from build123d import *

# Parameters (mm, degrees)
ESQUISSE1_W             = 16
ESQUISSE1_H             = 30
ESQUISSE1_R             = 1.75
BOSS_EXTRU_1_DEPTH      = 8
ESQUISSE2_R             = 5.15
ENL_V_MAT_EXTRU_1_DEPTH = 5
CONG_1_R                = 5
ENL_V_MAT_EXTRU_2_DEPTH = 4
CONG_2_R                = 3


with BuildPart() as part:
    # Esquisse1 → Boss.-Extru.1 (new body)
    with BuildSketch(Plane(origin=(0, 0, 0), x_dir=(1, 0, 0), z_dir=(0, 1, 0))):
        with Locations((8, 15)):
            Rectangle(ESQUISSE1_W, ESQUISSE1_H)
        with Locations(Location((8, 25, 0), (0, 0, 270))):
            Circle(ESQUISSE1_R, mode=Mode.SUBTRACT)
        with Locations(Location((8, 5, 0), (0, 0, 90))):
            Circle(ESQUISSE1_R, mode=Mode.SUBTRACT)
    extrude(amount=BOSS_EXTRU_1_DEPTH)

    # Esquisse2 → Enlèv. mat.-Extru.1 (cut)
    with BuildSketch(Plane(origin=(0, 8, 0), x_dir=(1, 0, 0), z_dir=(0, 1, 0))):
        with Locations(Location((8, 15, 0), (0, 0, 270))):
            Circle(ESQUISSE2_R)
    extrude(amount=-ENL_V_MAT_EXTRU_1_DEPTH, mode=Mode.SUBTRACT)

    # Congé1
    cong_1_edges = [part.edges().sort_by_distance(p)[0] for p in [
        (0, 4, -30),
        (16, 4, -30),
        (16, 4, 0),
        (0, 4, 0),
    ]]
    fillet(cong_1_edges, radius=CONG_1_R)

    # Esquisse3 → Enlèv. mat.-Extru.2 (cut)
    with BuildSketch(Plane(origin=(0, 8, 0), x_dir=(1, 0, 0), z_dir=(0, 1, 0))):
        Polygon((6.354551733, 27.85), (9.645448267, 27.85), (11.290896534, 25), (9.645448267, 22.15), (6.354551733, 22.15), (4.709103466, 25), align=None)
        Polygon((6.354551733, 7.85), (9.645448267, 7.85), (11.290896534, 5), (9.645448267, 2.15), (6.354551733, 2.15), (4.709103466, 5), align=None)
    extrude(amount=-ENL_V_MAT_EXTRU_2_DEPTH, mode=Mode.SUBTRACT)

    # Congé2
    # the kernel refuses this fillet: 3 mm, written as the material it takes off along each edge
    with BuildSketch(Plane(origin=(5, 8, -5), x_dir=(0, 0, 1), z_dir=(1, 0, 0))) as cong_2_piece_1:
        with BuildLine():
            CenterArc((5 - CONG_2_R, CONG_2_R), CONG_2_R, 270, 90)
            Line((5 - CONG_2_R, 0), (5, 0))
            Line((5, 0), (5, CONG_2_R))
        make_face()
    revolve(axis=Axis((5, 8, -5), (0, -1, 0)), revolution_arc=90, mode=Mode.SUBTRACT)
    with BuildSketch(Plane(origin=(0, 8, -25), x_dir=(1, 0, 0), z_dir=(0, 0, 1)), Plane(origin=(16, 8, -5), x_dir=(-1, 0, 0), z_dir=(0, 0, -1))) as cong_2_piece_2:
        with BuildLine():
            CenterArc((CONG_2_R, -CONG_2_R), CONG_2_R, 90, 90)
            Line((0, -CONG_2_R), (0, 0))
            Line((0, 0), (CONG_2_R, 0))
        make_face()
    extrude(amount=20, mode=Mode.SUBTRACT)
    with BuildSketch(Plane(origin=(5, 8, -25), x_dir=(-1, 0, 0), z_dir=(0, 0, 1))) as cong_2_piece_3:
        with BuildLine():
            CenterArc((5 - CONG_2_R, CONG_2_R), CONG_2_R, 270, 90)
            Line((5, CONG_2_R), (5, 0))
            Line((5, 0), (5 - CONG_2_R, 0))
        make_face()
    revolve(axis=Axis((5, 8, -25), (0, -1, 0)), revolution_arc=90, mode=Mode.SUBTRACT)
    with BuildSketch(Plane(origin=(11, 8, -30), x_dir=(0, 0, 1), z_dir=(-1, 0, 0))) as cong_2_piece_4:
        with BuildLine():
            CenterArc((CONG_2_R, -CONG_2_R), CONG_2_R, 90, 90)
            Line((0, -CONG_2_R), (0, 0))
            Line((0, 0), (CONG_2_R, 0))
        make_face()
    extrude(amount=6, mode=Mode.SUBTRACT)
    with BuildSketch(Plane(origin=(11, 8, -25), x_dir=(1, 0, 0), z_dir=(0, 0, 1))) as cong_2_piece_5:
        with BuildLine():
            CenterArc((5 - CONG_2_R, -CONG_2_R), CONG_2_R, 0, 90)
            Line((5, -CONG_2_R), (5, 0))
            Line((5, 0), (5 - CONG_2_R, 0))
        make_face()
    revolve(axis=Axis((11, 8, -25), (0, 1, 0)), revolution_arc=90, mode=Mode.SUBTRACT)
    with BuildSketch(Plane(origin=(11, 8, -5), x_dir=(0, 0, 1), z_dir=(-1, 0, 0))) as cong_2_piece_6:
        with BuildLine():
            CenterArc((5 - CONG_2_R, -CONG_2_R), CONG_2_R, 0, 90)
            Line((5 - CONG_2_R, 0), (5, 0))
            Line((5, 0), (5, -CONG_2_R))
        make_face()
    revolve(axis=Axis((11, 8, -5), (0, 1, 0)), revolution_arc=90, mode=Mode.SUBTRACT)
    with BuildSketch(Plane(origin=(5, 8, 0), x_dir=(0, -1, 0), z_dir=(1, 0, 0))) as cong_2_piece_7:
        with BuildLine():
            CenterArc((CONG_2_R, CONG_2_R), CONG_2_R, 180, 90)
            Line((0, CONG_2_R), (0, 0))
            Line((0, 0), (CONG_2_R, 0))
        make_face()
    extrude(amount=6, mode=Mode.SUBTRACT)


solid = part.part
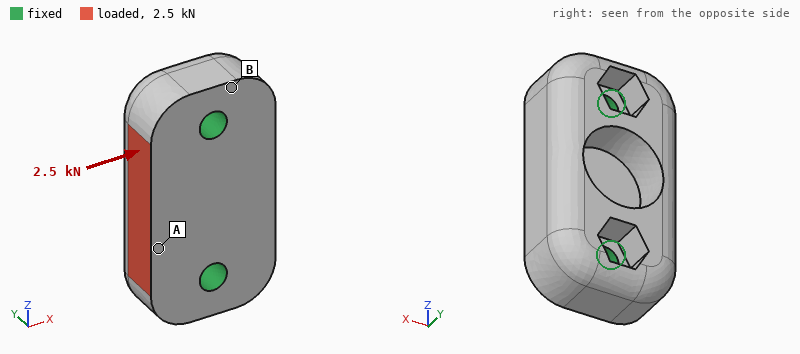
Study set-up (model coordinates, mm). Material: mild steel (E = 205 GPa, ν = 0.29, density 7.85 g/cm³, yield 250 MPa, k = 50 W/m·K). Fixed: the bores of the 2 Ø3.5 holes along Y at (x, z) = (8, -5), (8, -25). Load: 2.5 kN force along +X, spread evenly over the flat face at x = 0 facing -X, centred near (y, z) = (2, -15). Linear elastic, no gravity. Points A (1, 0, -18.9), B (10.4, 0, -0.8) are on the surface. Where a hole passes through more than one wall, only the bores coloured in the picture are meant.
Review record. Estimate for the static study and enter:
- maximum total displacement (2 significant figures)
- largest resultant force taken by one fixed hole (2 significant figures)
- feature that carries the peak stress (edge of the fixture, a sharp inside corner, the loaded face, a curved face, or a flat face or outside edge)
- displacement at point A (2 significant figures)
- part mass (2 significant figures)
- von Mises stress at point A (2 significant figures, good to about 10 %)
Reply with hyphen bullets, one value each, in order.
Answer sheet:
- 2.5 µm
- 1.3 kN
- edge of the fixture
- 1.8 µm
- 22 g
- 24 MPa
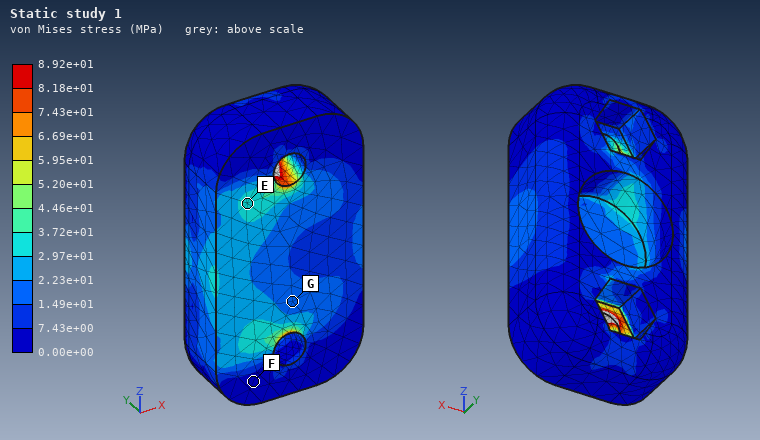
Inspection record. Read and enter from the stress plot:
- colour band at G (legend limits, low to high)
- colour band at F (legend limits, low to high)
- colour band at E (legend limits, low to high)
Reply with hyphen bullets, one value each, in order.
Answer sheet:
- 1.49e+01 to 2.23e+01 MPa
- 0.00e+00 to 7.43e+00 MPa
- 2.97e+01 to 3.72e+01 MPa
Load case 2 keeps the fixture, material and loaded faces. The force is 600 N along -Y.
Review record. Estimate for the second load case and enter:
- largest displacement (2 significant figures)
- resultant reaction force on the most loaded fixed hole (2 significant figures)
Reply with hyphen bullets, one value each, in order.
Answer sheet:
- 4.1 µm
- 300 N
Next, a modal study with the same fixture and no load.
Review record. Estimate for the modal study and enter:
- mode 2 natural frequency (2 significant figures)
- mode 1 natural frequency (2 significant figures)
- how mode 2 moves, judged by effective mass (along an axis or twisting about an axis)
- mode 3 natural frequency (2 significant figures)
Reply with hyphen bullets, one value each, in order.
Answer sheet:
- 39 kHz
- 28 kHz
- along Y
- 45 kHz
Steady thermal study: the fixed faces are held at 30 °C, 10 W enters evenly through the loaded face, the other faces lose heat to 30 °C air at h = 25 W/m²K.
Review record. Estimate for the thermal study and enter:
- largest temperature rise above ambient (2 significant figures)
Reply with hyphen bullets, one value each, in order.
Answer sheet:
- 17 K
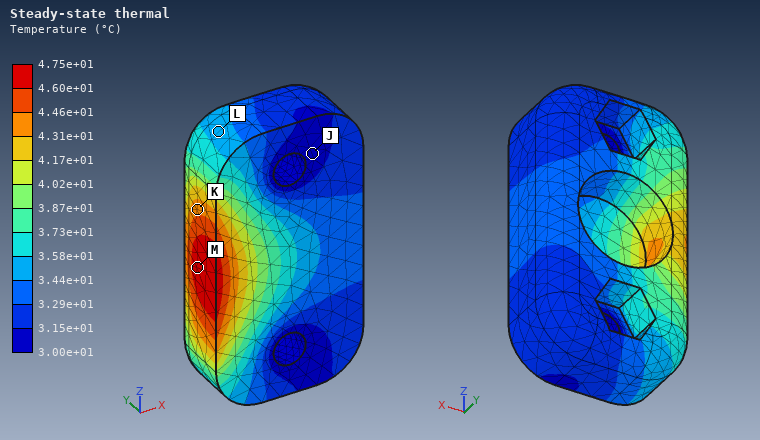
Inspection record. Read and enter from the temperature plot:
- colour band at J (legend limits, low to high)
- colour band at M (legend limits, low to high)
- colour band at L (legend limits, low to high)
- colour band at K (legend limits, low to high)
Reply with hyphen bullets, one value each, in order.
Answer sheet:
- 3.00e+01 to 3.15e+01 °C
- 4.60e+01 to 4.75e+01 °C
- 3.44e+01 to 3.58e+01 °C
- 4.31e+01 to 4.46e+01 °C
